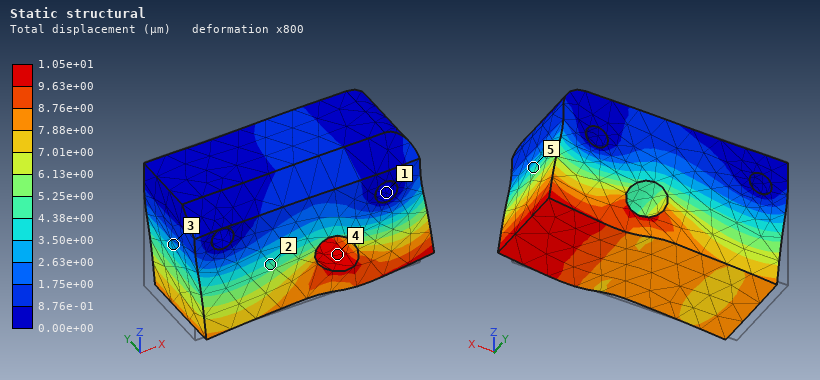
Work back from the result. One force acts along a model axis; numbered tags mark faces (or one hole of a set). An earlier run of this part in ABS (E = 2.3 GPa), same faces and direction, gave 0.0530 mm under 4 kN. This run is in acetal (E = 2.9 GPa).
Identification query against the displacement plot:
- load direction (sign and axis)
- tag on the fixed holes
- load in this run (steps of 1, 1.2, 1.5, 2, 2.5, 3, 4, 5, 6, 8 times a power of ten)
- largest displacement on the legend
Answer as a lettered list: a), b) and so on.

a) +X
b) 1
c) 1 kN
d) 1.05e+01 µm
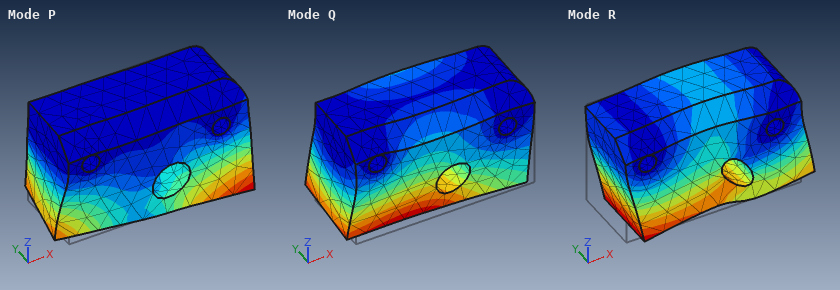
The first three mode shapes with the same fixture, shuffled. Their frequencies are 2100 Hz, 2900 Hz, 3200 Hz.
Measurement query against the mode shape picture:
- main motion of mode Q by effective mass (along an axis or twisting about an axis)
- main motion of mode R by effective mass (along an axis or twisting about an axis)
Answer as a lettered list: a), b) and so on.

a) along Y
b) along X
